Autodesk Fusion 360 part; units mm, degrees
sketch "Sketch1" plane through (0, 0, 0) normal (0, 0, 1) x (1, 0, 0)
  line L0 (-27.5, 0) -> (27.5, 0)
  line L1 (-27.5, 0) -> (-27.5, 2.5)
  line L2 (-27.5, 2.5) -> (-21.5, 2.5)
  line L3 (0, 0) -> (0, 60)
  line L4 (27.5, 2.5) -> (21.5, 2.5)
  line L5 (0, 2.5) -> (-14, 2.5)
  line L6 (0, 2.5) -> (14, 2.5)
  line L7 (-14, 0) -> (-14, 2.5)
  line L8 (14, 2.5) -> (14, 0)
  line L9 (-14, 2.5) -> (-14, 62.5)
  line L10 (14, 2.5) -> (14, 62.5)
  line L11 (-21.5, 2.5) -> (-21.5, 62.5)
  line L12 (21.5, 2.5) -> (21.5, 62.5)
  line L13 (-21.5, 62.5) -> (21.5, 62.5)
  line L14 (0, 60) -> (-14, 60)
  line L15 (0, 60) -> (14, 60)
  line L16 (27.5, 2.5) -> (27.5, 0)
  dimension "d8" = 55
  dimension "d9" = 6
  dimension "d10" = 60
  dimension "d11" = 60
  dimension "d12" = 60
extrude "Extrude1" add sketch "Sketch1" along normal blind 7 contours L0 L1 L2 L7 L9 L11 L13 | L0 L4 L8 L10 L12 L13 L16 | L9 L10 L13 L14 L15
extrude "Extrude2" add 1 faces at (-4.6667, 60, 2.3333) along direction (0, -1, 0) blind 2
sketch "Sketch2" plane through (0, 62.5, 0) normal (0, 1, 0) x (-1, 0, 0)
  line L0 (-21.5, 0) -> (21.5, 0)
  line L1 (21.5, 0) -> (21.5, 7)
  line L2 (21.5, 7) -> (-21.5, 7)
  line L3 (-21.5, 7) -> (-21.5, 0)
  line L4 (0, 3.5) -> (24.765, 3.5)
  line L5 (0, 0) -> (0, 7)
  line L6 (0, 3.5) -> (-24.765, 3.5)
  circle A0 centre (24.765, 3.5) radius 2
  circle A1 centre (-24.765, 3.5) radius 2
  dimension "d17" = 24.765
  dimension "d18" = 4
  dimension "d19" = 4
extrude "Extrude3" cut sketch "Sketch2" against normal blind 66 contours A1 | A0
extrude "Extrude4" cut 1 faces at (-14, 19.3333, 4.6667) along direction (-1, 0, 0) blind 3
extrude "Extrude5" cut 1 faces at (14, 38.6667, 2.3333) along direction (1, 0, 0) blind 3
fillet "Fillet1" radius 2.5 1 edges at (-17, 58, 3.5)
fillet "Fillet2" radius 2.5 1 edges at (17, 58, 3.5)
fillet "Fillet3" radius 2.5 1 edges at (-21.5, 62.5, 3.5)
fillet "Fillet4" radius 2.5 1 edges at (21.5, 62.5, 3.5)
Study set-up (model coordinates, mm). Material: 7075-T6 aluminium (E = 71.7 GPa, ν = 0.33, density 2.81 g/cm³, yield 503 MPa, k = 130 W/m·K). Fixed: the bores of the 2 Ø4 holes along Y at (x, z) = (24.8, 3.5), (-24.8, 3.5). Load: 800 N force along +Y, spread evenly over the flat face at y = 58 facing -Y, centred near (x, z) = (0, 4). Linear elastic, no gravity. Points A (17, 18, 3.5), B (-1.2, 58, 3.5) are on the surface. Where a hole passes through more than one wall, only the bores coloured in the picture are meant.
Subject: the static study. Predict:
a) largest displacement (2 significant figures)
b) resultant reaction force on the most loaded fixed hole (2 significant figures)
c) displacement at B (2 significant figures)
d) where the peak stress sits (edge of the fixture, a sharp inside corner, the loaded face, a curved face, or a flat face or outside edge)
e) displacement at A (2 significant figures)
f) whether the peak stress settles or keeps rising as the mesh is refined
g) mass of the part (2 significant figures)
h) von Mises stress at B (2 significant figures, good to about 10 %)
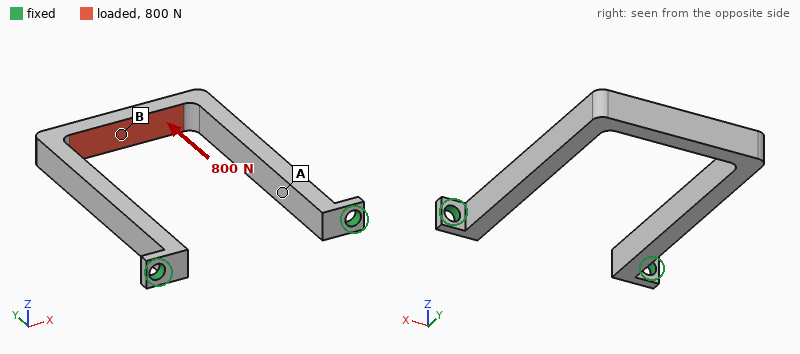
0.11 mm
400 N
0.11 mm
edge of the fixture
0.023 mm
keeps rising
14 g
110 MPa
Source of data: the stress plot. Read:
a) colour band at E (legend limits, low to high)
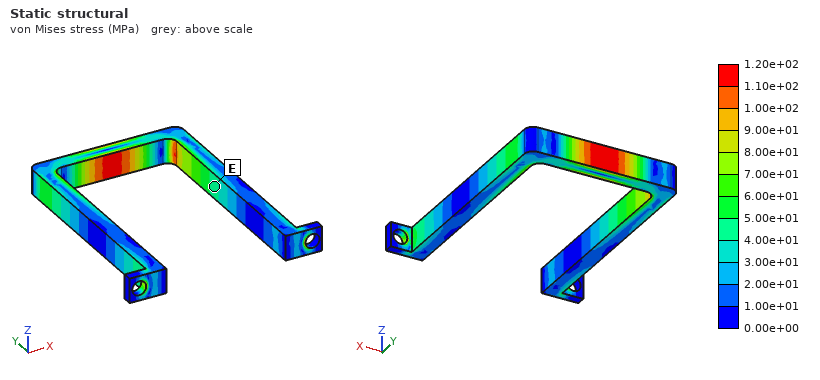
4.00e+01 to 5.00e+01 MPa
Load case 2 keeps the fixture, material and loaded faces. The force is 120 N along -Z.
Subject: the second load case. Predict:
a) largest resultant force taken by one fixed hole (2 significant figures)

60 N
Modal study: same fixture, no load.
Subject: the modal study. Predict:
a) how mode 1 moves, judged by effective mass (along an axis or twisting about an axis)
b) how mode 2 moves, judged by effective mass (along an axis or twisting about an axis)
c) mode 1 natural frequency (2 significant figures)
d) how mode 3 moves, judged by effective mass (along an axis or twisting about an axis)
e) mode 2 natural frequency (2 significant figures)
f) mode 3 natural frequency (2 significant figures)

along Z
along X
720 Hz
twisting about Y
930 Hz
1700 Hz
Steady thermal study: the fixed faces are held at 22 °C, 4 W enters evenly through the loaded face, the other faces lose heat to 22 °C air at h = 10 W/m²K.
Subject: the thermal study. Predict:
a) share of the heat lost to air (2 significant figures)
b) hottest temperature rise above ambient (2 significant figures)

15 %
32 K
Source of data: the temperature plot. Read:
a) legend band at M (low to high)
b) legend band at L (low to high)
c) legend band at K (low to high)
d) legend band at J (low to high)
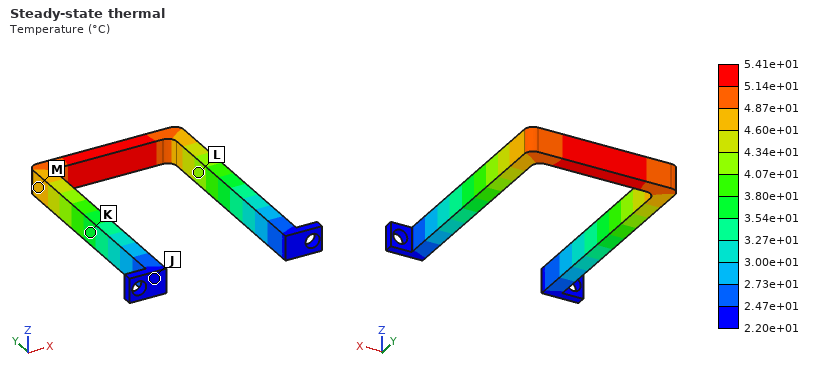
4.60e+01 to 4.87e+01 °C
4.07e+01 to 4.34e+01 °C
3.54e+01 to 3.80e+01 °C
2.20e+01 to 2.47e+01 °C
